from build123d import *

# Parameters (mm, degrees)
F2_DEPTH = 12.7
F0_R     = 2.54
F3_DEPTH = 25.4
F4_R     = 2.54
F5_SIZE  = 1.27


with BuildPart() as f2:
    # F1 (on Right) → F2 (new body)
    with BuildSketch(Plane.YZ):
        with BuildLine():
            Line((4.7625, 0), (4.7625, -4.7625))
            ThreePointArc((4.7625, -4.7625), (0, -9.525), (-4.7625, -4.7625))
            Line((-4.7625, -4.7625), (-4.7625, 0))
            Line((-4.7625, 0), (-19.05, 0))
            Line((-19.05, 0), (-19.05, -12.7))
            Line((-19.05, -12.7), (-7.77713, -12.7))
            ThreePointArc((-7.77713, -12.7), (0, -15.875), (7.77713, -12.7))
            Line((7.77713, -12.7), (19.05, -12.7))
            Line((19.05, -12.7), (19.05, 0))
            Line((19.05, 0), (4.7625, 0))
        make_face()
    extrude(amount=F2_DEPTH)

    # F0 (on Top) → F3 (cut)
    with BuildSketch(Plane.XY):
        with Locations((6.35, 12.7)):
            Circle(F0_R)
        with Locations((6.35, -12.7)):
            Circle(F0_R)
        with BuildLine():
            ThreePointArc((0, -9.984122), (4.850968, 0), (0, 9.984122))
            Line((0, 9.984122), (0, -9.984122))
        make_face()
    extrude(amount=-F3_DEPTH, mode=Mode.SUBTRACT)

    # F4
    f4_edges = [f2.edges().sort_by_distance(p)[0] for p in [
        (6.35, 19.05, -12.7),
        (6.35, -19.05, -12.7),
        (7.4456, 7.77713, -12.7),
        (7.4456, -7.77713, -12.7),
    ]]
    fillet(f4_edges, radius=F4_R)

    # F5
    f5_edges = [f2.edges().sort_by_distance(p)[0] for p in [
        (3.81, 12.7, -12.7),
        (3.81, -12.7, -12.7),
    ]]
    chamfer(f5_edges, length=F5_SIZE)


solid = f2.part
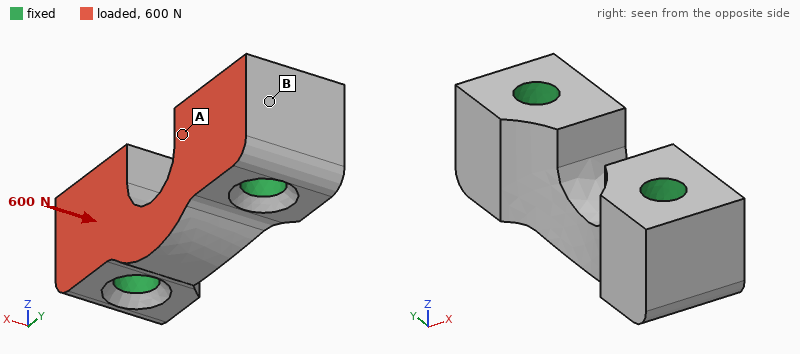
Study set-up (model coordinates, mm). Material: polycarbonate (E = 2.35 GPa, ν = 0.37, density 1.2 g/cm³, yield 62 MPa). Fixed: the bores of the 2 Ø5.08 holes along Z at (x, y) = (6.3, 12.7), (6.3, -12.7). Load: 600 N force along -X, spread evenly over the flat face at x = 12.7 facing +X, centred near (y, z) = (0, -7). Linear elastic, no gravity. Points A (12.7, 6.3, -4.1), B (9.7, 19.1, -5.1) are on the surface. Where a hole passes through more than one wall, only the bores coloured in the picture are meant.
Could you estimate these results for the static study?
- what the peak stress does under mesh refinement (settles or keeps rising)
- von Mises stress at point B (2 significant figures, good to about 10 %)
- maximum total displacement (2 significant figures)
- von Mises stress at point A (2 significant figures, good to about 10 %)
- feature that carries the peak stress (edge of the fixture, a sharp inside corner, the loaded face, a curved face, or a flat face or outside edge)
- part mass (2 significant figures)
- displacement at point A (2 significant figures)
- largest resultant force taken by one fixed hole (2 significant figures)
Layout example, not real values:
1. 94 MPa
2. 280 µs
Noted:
1. keeps rising
2. 1.0 MPa
3. 34 µm
4. 2.0 MPa
5. edge of the fixture
6. 5.2 g
7. 12 µm
8. 300 N
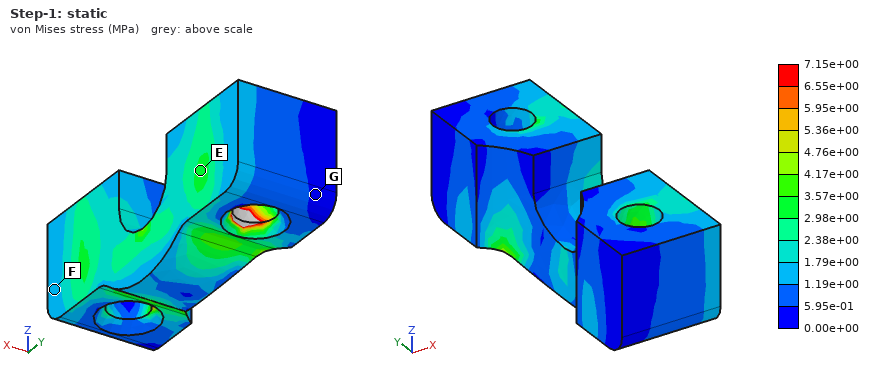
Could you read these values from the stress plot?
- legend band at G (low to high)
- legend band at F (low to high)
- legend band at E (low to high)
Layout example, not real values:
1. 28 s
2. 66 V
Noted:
1. 0.00e+00 to 5.95e-01 MPa
2. 1.19e+00 to 1.79e+00 MPa
3. 2.98e+00 to 3.57e+00 MPa
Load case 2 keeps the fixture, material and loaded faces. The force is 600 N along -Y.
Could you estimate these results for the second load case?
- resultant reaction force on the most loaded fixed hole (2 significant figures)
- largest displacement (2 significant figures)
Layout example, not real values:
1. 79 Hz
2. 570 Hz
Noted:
1. 310 N
2. 24 µm
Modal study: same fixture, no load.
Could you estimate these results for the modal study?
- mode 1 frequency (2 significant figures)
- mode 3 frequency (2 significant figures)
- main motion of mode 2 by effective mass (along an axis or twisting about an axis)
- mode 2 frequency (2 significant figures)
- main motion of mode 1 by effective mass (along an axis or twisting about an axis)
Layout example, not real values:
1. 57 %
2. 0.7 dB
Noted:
1. 13 kHz
2. 21 kHz
3. along Z
4. 19 kHz
5. along X
